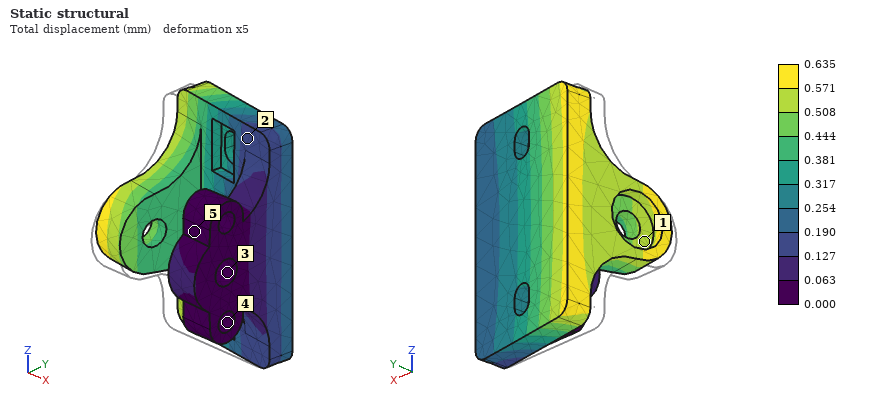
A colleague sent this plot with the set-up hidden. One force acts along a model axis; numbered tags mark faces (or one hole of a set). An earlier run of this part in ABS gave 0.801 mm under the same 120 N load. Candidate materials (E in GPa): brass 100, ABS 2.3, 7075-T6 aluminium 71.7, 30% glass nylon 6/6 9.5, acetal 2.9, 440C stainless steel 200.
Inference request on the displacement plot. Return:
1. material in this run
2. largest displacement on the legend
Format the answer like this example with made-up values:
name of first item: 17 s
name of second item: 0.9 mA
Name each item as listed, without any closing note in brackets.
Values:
material in this run: acetal
largest displacement on the legend: 0.635 mm
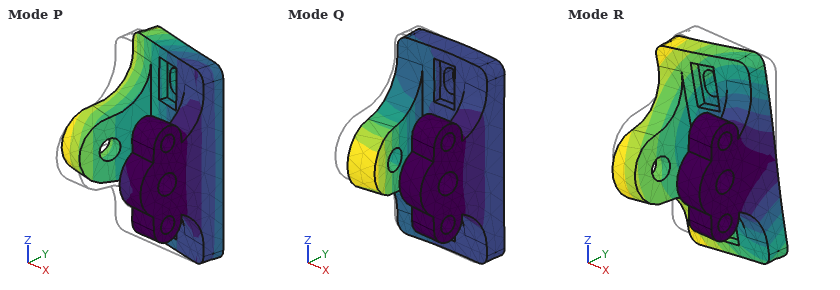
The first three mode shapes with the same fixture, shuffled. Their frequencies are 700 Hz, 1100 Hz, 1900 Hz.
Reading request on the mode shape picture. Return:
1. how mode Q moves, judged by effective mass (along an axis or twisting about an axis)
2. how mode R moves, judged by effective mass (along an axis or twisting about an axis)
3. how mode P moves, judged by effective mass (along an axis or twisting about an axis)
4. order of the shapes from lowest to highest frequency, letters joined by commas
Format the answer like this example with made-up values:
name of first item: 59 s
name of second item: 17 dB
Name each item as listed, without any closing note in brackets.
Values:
how mode Q moves, judged by effective mass: along X
how mode R moves, judged by effective mass: along Z
how mode P moves, judged by effective mass: along Y
order of the shapes from lowest to highest frequency, letters joined by commas: P, R, Q
